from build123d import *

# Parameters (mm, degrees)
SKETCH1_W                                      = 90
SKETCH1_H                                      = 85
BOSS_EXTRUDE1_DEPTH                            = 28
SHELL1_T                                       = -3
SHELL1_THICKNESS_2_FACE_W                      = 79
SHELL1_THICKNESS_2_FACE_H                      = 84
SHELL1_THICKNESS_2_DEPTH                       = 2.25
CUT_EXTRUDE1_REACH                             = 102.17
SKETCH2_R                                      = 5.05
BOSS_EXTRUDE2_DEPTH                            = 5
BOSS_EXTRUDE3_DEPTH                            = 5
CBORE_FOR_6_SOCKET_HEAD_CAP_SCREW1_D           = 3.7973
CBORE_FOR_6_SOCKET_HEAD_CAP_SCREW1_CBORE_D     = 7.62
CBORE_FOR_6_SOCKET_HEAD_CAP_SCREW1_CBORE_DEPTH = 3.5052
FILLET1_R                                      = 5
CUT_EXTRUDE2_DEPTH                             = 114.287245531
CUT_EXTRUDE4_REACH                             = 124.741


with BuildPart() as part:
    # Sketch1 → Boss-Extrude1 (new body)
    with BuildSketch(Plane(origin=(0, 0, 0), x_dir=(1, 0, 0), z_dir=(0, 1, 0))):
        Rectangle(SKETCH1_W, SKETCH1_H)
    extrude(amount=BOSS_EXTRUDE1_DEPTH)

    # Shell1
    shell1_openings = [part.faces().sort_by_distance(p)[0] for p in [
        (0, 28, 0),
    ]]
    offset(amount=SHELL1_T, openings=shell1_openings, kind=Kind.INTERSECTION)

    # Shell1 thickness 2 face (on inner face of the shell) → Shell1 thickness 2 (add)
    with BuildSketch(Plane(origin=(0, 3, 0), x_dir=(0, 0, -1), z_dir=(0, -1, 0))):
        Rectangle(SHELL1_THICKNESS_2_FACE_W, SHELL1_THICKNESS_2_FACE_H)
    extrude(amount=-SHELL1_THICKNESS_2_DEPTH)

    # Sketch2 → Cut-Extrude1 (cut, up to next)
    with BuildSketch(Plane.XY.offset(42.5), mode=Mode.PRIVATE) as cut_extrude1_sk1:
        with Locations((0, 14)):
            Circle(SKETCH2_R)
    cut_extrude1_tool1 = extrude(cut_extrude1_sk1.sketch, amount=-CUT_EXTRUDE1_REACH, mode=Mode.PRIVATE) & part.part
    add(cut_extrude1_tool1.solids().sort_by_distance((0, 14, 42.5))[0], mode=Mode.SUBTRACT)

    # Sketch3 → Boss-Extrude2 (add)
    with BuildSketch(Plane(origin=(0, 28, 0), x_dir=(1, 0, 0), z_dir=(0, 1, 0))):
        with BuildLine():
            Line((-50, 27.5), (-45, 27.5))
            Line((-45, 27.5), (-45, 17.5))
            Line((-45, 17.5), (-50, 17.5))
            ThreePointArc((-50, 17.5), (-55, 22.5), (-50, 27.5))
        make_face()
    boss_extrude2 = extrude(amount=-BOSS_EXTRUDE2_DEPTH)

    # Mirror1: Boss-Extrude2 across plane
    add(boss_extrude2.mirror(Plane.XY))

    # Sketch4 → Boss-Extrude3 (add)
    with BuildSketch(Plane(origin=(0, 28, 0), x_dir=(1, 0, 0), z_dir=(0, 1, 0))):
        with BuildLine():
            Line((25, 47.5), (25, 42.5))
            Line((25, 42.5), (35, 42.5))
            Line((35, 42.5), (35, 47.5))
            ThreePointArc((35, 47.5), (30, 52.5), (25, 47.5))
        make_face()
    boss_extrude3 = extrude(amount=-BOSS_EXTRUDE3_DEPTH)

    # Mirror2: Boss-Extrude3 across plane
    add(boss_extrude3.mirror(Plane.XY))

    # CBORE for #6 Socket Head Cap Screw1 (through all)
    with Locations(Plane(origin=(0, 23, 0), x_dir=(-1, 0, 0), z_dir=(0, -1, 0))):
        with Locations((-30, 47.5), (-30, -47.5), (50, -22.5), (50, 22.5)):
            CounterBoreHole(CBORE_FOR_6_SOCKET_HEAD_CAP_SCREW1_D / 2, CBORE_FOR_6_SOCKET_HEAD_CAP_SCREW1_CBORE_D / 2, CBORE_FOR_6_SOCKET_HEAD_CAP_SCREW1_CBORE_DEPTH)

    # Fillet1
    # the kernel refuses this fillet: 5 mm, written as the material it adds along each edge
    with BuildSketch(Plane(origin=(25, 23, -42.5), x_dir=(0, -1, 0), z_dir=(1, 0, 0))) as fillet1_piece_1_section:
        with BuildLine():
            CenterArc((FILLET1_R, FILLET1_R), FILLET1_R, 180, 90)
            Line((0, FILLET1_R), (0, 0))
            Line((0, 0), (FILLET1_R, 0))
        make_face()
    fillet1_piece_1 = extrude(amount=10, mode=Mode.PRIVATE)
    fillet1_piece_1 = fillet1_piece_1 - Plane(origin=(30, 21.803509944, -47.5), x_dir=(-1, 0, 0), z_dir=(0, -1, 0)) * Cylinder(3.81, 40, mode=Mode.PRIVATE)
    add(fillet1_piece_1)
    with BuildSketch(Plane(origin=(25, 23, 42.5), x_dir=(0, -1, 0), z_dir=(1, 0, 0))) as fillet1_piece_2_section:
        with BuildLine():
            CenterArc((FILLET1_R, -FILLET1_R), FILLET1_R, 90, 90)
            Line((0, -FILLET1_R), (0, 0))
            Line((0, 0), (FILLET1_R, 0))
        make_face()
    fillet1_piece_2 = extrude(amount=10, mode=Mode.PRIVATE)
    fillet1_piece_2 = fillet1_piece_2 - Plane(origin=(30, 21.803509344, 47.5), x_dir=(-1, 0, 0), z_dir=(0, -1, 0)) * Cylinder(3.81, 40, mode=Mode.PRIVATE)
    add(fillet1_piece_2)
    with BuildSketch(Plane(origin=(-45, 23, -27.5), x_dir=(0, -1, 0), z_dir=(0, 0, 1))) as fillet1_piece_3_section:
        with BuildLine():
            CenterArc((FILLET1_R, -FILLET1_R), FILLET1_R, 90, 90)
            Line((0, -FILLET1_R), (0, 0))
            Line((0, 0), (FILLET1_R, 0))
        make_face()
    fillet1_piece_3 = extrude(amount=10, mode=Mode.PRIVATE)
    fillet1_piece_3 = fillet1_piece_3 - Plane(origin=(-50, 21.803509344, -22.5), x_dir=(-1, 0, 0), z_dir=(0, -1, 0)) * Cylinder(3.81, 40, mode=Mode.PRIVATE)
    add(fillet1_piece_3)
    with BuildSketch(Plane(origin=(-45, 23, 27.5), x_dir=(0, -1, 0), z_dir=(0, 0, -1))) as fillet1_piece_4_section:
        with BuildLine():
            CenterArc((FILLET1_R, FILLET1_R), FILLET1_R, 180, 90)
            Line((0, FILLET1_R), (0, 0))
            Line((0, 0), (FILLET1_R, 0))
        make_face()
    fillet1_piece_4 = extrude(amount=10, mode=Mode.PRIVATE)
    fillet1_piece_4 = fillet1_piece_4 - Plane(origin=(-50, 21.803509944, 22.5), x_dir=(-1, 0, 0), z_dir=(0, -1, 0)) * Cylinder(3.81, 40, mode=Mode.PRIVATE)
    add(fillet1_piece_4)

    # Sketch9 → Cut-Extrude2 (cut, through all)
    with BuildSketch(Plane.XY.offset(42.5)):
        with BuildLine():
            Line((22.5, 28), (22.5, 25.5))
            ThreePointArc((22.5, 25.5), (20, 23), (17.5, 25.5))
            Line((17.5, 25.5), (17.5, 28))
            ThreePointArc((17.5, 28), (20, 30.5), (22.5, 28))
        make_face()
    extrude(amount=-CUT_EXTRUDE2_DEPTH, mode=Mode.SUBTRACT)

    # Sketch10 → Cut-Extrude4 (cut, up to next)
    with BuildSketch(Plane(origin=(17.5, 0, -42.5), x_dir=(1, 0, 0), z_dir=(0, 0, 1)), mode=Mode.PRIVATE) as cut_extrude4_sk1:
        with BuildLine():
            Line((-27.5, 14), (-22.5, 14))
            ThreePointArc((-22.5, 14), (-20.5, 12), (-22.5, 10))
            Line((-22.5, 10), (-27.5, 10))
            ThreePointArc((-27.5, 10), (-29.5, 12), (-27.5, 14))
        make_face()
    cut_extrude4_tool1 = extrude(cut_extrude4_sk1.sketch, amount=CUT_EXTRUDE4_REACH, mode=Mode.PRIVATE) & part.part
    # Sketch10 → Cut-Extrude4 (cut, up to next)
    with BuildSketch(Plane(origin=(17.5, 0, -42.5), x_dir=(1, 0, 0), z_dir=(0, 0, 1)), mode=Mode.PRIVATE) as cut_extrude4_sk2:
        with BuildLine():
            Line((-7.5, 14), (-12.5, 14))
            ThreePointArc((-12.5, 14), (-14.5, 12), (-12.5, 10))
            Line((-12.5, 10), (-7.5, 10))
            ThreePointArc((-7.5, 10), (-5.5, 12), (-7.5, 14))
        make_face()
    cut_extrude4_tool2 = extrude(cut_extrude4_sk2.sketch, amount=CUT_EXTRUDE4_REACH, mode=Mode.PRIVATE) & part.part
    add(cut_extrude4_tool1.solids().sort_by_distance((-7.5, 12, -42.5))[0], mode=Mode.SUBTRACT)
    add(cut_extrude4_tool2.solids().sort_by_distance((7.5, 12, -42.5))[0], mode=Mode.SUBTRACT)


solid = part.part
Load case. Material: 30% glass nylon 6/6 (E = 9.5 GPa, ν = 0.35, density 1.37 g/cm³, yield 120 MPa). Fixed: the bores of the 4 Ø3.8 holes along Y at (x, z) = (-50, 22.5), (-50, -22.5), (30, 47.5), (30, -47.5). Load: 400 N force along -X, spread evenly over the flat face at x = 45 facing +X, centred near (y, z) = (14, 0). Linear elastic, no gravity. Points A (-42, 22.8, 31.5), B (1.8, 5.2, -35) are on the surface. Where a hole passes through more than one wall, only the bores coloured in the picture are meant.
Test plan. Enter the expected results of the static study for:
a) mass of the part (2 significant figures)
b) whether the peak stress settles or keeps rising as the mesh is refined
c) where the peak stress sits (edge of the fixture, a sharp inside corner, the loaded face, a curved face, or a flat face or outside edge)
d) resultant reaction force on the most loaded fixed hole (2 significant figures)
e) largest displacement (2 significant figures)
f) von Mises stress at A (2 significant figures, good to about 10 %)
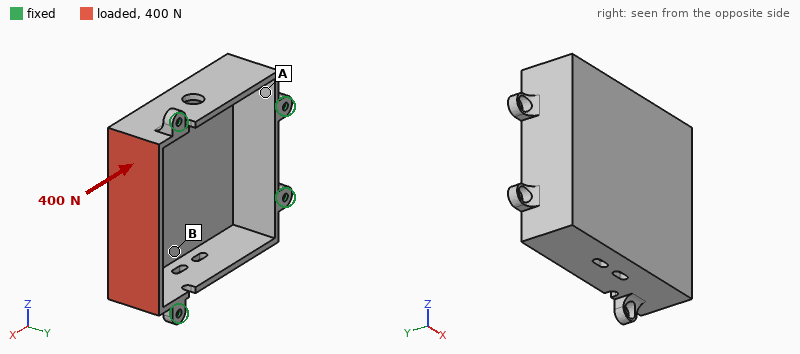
88 g
keeps rising
edge of the fixture
170 N
0.29 mm
3.2 MPa
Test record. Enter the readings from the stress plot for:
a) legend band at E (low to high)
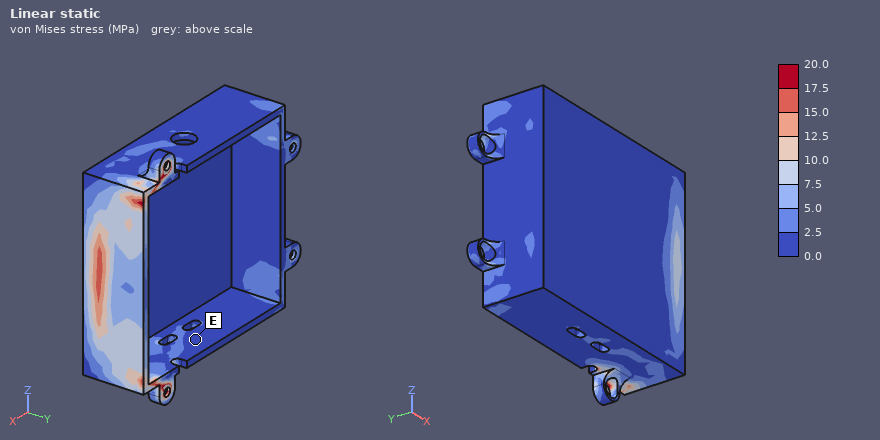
0.0 to 2.5 MPa
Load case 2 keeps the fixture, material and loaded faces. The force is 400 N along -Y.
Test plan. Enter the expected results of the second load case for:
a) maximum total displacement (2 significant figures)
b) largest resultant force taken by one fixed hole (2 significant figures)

0.13 mm
260 N
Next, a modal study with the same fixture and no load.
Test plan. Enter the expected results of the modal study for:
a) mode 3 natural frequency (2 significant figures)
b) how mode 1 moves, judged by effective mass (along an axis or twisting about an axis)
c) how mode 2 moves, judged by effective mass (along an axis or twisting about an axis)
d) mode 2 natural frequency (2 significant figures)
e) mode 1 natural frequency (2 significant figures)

1800 Hz
along Z
along X
1500 Hz
1400 Hz
